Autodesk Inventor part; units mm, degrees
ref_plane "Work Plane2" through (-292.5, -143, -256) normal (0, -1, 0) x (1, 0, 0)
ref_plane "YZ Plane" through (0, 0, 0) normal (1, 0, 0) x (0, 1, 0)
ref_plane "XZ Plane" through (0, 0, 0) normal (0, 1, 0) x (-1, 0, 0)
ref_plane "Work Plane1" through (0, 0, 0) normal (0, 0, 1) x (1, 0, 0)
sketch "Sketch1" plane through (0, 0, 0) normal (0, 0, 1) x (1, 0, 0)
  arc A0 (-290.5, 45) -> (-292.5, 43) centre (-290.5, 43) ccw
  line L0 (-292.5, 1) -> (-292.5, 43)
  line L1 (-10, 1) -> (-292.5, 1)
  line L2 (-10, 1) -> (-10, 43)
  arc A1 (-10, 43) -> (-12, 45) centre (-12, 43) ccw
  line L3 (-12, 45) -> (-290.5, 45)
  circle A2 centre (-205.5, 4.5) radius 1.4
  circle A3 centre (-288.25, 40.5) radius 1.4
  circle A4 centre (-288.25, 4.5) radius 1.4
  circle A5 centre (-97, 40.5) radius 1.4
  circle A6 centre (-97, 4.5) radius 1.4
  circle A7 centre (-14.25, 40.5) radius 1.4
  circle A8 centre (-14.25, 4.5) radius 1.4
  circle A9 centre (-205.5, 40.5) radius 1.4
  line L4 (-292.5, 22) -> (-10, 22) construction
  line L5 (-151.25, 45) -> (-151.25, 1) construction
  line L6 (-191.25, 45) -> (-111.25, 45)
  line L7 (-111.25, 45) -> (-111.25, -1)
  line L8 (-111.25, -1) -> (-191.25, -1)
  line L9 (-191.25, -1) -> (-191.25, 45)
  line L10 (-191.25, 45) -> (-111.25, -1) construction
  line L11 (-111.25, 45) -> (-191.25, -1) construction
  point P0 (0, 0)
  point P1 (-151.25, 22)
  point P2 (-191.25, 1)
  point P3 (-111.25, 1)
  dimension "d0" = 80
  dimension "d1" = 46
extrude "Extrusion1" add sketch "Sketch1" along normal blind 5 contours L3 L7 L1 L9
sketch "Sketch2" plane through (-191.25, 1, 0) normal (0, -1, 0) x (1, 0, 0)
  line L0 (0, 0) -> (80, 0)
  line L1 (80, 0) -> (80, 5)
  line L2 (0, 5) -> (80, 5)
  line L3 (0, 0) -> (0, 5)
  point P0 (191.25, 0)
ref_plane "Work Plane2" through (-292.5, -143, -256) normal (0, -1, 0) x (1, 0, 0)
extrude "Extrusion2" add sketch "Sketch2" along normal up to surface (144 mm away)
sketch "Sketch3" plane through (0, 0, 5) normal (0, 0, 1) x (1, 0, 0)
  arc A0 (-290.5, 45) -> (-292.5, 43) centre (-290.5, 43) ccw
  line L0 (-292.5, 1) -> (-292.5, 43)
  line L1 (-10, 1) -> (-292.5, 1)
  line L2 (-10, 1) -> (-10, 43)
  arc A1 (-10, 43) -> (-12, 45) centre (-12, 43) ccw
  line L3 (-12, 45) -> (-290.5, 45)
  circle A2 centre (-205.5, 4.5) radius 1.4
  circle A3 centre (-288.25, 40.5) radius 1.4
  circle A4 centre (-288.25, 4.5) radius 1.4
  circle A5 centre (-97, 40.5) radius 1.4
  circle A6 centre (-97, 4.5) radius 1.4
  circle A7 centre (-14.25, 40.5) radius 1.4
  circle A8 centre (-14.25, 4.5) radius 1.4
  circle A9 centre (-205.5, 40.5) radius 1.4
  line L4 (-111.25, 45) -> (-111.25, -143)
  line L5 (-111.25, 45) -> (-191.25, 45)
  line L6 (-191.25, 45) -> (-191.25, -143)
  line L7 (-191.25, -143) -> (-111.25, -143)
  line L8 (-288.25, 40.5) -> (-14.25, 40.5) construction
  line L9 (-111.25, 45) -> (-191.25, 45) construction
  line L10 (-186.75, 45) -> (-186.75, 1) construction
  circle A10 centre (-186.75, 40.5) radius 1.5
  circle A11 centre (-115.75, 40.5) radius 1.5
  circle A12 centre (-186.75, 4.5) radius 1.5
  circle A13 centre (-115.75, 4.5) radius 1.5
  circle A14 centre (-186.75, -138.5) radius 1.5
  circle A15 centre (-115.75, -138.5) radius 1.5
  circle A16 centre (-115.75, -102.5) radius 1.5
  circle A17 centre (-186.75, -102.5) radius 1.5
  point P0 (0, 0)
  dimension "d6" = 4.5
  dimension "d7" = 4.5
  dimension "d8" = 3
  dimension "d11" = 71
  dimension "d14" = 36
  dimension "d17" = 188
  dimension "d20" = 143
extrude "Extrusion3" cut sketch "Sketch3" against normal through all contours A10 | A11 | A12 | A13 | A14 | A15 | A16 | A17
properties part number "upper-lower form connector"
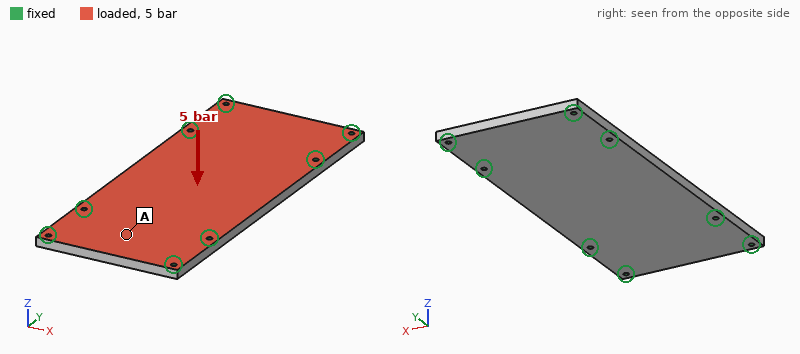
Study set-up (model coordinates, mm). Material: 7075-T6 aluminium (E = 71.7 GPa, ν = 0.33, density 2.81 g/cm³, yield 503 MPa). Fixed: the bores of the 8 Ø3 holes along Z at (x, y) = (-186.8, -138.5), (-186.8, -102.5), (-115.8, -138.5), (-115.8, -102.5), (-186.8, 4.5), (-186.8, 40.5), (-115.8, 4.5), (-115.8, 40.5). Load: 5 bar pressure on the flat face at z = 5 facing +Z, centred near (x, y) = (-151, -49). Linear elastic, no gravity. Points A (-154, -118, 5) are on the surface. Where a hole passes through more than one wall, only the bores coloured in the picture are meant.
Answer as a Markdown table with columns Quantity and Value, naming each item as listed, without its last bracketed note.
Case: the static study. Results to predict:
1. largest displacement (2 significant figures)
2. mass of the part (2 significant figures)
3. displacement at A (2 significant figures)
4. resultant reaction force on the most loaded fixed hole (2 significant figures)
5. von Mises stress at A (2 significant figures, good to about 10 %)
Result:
| Quantity | Value |
|---|---|
| largest displacement | 0.37 mm |
| mass of the part | 210 g |
| displacement at A | 0.069 mm |
| resultant reaction force on the most loaded fixed hole | 1.6 kN |
| von Mises stress at A | 35 MPa |
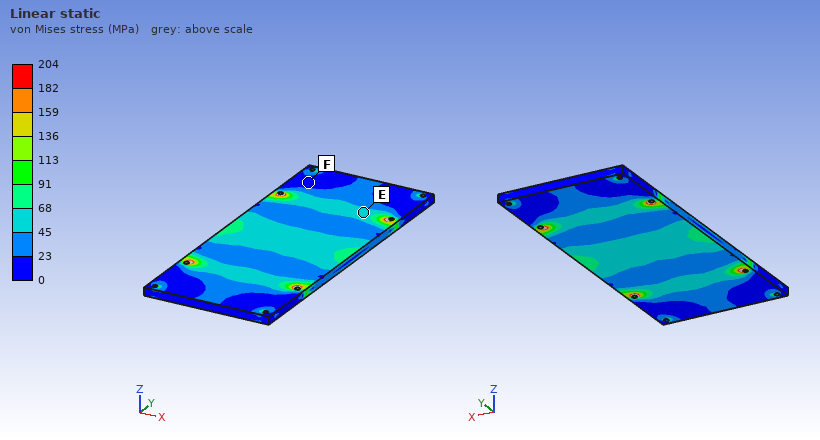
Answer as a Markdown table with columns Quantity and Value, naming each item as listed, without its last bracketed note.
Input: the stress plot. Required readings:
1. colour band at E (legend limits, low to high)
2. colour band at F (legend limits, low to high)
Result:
| Quantity | Value |
|---|---|
| colour band at E | 45 to 68 MPa |
| colour band at F | 0 to 23 MPa |
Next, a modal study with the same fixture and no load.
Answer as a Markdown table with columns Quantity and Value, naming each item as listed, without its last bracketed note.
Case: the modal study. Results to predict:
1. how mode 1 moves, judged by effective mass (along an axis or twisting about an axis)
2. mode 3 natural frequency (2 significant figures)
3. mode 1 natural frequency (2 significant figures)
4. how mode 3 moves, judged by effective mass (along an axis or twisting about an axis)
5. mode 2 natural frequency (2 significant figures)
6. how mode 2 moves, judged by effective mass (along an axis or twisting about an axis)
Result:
| Quantity | Value |
|---|---|
| how mode 1 moves, judged by effective mass | along Z |
| mode 3 natural frequency | 4100 Hz |
| mode 1 natural frequency | 1800 Hz |
| how mode 3 moves, judged by effective mass | twisting about X |
| mode 2 natural frequency | 2900 Hz |
| how mode 2 moves, judged by effective mass | twisting about Y |
